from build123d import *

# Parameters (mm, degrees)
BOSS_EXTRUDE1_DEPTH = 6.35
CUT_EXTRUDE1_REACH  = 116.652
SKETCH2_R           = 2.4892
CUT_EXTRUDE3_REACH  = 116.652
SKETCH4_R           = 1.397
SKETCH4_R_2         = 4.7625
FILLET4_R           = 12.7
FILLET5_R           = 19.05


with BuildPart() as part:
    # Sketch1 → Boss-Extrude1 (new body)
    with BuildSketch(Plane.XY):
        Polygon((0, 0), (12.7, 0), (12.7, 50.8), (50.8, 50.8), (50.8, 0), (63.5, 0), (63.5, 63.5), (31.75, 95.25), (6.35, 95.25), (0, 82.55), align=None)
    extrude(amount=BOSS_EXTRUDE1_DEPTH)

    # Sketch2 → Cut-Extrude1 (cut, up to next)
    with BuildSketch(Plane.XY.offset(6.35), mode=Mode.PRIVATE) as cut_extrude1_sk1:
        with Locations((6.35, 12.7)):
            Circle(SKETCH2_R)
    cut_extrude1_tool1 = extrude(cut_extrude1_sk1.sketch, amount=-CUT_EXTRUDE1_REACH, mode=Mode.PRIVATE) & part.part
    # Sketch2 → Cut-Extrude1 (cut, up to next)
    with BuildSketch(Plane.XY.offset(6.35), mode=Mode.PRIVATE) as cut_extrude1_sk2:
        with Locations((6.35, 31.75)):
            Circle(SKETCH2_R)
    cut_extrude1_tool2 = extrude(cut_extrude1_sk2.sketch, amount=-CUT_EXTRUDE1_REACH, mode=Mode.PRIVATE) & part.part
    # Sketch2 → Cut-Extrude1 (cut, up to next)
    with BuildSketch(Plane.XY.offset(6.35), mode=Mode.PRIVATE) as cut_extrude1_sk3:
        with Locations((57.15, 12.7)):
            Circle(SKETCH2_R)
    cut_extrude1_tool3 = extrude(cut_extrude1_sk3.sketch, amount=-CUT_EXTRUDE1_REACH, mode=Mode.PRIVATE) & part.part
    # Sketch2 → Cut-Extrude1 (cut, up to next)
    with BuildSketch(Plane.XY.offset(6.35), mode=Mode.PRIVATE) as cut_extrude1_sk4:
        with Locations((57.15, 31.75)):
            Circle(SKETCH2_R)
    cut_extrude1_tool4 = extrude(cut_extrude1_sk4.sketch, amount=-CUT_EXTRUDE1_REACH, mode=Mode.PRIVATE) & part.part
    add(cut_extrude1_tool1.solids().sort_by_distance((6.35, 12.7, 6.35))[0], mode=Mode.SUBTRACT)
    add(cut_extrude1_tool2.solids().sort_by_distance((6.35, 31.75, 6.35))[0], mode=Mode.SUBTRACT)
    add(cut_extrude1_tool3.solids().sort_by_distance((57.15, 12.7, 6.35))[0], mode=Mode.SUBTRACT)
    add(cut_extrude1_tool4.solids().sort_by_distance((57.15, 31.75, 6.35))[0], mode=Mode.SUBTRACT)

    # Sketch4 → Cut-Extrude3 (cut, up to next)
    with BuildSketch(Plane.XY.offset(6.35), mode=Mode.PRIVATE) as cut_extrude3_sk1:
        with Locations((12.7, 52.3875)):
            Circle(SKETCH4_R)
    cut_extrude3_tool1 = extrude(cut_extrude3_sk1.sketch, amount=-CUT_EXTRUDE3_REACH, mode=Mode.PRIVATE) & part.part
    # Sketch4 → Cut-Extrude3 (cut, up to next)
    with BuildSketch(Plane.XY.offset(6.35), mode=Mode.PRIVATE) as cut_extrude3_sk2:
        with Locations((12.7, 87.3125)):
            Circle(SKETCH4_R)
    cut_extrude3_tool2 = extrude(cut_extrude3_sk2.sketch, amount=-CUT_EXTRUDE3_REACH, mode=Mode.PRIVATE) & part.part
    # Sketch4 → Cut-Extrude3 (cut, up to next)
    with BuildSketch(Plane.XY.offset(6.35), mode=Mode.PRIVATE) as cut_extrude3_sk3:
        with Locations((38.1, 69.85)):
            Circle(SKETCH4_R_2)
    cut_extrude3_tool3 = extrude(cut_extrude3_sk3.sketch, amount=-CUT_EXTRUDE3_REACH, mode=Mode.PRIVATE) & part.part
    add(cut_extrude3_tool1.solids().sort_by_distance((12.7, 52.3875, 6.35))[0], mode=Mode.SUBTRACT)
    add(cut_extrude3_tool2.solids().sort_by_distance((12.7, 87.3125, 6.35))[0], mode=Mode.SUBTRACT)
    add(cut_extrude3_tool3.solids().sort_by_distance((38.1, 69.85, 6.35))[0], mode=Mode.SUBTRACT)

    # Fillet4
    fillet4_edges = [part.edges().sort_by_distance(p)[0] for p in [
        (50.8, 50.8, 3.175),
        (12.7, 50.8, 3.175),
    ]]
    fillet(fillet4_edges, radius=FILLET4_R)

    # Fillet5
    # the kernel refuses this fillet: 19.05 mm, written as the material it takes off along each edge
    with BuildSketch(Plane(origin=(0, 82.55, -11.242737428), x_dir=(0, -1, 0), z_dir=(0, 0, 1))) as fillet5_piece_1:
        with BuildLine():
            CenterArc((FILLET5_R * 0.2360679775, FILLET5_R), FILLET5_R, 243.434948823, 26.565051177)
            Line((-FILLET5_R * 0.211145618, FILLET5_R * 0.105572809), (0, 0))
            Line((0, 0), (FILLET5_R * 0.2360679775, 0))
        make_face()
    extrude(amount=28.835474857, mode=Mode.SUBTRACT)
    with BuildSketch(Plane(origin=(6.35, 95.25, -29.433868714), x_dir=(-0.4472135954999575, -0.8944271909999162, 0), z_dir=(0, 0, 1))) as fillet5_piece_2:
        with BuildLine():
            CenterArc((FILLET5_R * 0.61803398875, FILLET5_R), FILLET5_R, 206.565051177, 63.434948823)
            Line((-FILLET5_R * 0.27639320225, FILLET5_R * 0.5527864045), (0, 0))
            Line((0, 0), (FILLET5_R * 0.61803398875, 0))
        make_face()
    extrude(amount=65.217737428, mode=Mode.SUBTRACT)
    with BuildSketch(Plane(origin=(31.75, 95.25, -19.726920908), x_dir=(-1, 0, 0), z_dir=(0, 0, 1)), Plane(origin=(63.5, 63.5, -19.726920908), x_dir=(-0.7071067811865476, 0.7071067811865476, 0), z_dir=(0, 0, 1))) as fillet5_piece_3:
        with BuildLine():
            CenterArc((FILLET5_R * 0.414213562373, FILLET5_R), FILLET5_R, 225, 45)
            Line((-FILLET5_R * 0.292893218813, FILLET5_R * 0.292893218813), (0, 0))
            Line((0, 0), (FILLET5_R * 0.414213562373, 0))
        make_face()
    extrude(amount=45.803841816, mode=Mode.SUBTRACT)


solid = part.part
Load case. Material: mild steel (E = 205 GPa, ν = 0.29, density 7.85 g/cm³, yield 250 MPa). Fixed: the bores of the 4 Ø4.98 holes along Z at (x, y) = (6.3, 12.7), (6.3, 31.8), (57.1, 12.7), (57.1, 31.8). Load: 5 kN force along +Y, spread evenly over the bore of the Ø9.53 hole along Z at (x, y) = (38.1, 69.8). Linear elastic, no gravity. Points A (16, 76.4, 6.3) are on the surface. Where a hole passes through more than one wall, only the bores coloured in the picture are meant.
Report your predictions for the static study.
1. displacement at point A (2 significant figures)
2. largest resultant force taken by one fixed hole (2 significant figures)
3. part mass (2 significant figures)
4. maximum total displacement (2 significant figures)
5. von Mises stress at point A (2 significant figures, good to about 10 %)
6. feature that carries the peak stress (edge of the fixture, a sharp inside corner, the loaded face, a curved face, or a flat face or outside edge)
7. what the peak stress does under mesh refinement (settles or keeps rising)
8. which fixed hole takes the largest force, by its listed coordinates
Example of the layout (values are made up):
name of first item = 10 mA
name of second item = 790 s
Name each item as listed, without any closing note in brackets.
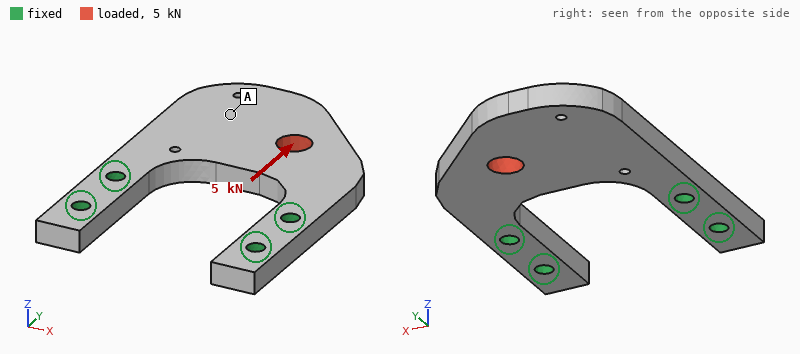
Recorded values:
displacement at point A = 4.3 µm
largest resultant force taken by one fixed hole = 3.1 kN
part mass = 170 g
maximum total displacement = 8.7 µm
von Mises stress at point A = 7.7 MPa
feature that carries the peak stress = edge of the fixture
what the peak stress does under mesh refinement = keeps rising
which fixed hole takes the largest force, by its listed coordinates = (57.1, 31.8)
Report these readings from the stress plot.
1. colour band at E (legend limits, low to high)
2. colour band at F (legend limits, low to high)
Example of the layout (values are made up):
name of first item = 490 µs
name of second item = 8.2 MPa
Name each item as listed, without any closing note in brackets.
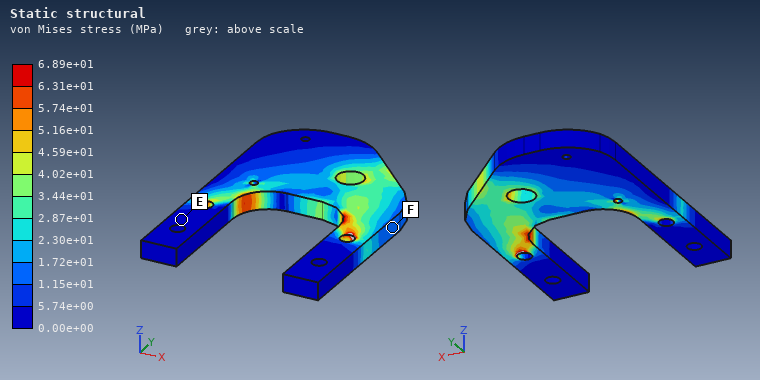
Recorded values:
colour band at E = 0.00e+00 to 5.74e+00 MPa
colour band at F = 1.15e+01 to 1.72e+01 MPa
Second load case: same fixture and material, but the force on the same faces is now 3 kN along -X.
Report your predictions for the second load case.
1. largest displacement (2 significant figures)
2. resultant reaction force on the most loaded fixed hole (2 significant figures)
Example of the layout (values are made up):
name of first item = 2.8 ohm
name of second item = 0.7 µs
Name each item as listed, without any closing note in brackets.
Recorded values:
largest displacement = 16 µm
resultant reaction force on the most loaded fixed hole = 2.4 kN
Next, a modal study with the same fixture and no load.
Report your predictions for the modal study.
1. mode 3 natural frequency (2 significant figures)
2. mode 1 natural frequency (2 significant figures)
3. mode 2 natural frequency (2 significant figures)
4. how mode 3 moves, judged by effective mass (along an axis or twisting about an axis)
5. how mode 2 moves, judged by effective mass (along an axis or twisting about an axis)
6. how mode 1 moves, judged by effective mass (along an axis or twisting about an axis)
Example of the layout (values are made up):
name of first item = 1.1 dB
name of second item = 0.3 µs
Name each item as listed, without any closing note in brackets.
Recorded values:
mode 3 natural frequency = 6900 Hz
mode 1 natural frequency = 1100 Hz
mode 2 natural frequency = 4000 Hz
how mode 3 moves, judged by effective mass = along X
how mode 2 moves, judged by effective mass = twisting about Y
how mode 1 moves, judged by effective mass = along Z
